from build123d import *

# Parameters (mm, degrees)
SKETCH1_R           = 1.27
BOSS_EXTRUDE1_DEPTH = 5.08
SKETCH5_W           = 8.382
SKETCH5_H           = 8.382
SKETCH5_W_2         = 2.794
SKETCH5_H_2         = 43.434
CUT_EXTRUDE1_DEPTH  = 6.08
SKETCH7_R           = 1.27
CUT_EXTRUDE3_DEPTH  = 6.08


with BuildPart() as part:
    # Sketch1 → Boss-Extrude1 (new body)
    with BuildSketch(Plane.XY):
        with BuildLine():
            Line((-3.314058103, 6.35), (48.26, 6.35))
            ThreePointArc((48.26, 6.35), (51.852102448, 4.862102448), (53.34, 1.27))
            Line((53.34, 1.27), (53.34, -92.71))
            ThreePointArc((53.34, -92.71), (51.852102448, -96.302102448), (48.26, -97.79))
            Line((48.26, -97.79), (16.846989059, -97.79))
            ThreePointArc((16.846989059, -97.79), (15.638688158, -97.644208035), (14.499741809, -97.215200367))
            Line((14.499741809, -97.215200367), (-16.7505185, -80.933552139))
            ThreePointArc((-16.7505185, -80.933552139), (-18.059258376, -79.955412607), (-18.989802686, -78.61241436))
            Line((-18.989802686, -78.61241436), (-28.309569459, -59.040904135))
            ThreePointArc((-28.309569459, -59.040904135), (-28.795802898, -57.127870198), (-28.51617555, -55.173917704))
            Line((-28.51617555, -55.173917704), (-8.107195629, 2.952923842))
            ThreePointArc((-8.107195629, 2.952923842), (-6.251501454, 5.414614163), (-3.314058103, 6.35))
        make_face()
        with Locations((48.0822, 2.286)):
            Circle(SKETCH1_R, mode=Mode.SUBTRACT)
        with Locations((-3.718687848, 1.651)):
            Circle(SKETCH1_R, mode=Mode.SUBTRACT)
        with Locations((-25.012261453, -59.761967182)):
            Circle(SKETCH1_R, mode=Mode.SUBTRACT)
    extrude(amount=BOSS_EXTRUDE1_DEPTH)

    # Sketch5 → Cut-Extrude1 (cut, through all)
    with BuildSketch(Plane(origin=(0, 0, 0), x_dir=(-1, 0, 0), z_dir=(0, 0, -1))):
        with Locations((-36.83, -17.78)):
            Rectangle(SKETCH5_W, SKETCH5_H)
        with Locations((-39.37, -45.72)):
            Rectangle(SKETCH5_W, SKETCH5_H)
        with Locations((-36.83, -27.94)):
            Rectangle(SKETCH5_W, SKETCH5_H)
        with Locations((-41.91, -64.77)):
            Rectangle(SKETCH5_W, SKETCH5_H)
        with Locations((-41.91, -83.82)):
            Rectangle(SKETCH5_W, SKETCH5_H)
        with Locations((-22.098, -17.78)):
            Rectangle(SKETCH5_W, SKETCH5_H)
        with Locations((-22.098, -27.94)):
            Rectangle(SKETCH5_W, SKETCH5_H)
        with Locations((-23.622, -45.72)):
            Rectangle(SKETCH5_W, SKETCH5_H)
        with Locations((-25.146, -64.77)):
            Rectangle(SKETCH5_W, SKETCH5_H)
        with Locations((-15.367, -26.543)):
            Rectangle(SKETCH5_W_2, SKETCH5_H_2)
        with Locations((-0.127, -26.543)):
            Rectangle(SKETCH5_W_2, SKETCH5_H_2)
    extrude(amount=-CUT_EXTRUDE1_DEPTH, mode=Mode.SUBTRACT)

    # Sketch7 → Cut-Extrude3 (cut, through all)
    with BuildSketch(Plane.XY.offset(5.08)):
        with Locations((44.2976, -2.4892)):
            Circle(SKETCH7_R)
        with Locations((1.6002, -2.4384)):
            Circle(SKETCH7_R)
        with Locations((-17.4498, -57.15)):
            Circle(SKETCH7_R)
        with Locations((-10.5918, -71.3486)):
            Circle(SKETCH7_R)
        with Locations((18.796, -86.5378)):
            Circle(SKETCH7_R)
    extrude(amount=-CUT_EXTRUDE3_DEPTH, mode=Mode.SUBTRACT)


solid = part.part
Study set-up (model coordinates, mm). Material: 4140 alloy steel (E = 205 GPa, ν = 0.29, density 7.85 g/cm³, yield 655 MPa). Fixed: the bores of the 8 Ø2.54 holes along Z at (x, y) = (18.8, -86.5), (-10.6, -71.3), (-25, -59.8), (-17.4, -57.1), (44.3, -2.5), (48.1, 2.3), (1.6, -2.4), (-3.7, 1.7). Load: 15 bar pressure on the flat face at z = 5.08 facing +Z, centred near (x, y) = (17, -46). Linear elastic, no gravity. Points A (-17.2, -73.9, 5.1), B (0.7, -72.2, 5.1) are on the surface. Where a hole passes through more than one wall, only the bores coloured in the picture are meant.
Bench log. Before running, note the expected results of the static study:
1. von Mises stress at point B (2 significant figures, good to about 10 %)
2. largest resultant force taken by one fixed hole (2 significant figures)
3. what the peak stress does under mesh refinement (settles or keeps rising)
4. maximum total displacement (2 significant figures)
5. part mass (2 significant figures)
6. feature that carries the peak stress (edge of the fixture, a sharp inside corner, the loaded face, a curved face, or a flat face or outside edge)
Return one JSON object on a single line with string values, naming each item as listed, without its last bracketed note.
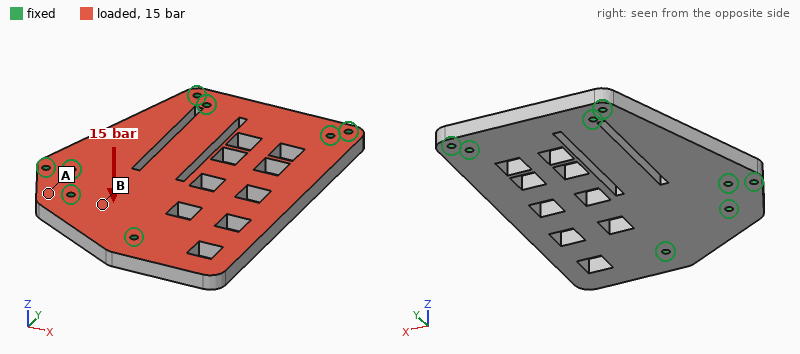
{"von Mises stress at point B": "76 MPa", "largest resultant force taken by one fixed hole": "3.3 kN", "what the peak stress does under mesh refinement": "keeps rising", "maximum total displacement": "0.23 mm", "part mass": "250 g", "feature that carries the peak stress": "edge of the fixture"}
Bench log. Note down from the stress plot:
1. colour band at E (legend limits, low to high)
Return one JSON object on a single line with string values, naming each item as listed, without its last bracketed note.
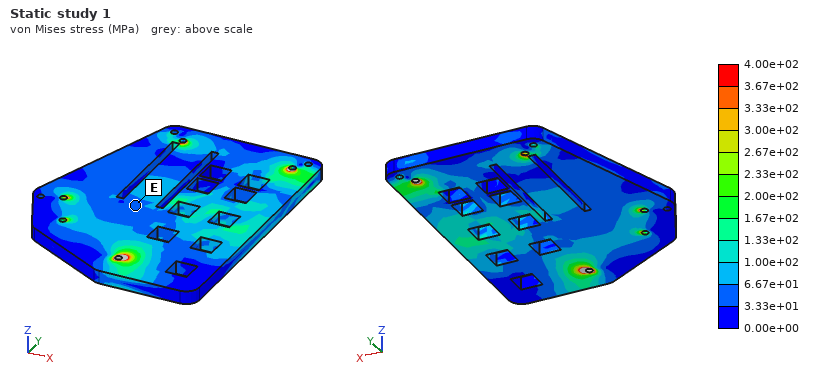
{"colour band at E": "3.33e+01 to 6.67e+01 MPa"}
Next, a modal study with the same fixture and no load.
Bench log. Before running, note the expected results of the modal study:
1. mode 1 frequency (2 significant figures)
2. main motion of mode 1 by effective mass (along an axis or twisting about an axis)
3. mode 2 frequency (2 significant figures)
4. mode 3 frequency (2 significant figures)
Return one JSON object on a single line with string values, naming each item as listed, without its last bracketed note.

{"mode 1 frequency": "2600 Hz", "main motion of mode 1 by effective mass": "along Z", "mode 2 frequency": "4300 Hz", "mode 3 frequency": "5900 Hz"}
